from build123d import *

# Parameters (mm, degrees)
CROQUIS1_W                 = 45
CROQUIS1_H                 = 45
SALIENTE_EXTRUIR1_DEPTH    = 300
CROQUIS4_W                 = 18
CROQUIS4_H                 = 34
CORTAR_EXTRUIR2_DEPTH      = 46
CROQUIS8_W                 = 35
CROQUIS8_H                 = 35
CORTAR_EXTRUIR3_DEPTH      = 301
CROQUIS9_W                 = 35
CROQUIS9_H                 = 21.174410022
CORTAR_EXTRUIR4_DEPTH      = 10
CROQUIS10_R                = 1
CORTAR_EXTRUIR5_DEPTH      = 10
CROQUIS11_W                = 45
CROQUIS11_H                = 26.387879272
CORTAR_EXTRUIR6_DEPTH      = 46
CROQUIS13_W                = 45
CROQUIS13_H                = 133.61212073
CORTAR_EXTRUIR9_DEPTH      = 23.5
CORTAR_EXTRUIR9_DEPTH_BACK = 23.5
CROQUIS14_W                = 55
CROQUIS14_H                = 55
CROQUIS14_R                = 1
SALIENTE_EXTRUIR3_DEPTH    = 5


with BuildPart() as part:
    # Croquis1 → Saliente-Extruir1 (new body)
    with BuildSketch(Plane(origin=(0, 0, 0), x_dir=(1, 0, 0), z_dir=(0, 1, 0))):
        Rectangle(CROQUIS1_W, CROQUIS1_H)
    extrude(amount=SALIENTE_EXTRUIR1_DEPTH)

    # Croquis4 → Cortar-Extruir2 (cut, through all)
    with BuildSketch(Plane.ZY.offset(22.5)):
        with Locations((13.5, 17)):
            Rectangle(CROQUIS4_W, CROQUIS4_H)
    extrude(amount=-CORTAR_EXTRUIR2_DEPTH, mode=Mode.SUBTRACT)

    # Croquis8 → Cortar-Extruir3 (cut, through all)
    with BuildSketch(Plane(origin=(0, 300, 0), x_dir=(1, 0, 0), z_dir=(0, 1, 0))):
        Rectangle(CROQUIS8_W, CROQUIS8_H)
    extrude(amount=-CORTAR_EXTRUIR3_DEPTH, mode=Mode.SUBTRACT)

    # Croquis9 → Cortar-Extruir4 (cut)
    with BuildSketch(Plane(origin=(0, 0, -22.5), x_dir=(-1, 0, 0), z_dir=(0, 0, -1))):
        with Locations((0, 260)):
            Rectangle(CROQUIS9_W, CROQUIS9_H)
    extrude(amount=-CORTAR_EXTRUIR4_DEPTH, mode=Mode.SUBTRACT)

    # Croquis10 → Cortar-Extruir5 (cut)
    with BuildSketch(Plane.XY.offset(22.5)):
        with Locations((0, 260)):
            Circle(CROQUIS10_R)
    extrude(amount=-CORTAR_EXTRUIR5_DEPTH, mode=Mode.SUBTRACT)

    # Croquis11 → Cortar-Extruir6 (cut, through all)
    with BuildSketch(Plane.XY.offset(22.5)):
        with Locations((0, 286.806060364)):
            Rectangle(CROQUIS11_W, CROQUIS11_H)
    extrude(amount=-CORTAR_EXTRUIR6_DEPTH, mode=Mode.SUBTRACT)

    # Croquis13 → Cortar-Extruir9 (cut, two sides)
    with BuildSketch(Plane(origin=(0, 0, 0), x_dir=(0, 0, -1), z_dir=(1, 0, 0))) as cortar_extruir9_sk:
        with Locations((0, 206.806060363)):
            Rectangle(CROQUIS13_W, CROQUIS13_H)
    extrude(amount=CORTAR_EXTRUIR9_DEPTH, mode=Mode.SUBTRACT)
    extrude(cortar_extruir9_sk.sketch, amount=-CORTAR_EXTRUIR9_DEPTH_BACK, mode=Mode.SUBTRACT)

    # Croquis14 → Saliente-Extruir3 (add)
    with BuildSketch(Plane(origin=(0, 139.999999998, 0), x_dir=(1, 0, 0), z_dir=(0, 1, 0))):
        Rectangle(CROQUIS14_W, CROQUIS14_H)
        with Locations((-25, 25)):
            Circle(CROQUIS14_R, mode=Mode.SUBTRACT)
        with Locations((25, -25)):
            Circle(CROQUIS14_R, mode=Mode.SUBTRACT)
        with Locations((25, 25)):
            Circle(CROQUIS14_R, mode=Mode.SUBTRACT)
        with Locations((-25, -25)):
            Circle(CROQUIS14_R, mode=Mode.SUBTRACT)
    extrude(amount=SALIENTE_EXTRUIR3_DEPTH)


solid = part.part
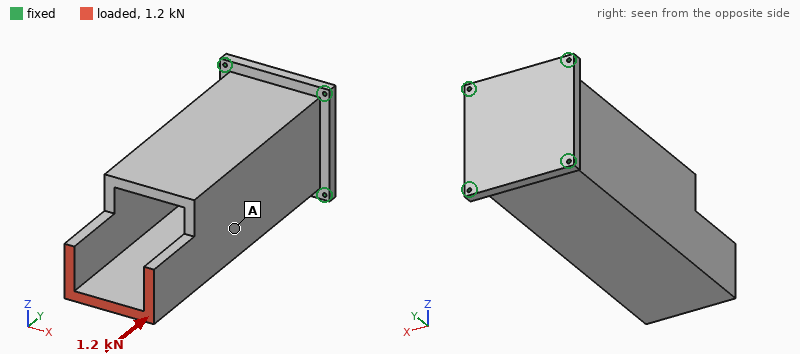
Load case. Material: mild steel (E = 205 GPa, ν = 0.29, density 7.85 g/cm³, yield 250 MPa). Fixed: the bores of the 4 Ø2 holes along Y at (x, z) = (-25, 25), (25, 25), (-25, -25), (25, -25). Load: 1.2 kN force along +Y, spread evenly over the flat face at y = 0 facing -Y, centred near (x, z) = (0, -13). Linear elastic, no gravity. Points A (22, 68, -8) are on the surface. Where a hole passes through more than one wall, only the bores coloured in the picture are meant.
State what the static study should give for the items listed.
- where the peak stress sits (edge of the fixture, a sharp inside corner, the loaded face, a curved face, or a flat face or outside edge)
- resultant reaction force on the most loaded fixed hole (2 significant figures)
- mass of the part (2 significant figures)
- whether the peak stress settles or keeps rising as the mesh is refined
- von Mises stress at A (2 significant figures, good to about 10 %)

edge of the fixture
490 N
900 g
keeps rising
2.1 MPa
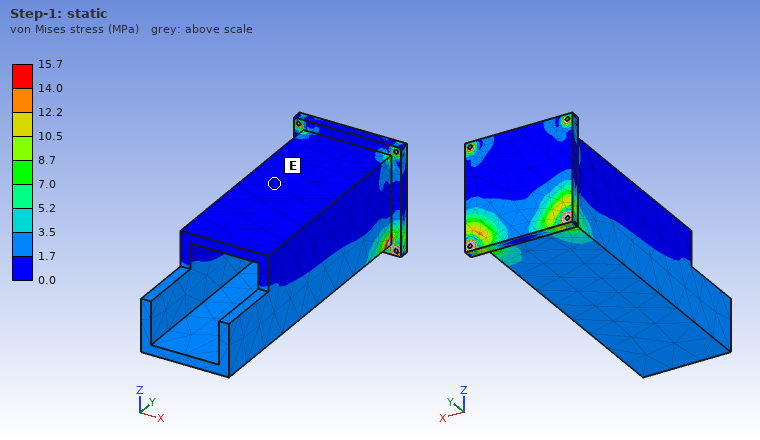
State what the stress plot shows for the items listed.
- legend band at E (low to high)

0.0 to 1.7 MPa
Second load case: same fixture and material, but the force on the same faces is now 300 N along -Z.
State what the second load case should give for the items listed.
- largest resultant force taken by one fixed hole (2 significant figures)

480 N
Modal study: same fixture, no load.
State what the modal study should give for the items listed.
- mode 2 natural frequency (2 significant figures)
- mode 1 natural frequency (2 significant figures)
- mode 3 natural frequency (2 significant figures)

1300 Hz
1300 Hz
4000 Hz
